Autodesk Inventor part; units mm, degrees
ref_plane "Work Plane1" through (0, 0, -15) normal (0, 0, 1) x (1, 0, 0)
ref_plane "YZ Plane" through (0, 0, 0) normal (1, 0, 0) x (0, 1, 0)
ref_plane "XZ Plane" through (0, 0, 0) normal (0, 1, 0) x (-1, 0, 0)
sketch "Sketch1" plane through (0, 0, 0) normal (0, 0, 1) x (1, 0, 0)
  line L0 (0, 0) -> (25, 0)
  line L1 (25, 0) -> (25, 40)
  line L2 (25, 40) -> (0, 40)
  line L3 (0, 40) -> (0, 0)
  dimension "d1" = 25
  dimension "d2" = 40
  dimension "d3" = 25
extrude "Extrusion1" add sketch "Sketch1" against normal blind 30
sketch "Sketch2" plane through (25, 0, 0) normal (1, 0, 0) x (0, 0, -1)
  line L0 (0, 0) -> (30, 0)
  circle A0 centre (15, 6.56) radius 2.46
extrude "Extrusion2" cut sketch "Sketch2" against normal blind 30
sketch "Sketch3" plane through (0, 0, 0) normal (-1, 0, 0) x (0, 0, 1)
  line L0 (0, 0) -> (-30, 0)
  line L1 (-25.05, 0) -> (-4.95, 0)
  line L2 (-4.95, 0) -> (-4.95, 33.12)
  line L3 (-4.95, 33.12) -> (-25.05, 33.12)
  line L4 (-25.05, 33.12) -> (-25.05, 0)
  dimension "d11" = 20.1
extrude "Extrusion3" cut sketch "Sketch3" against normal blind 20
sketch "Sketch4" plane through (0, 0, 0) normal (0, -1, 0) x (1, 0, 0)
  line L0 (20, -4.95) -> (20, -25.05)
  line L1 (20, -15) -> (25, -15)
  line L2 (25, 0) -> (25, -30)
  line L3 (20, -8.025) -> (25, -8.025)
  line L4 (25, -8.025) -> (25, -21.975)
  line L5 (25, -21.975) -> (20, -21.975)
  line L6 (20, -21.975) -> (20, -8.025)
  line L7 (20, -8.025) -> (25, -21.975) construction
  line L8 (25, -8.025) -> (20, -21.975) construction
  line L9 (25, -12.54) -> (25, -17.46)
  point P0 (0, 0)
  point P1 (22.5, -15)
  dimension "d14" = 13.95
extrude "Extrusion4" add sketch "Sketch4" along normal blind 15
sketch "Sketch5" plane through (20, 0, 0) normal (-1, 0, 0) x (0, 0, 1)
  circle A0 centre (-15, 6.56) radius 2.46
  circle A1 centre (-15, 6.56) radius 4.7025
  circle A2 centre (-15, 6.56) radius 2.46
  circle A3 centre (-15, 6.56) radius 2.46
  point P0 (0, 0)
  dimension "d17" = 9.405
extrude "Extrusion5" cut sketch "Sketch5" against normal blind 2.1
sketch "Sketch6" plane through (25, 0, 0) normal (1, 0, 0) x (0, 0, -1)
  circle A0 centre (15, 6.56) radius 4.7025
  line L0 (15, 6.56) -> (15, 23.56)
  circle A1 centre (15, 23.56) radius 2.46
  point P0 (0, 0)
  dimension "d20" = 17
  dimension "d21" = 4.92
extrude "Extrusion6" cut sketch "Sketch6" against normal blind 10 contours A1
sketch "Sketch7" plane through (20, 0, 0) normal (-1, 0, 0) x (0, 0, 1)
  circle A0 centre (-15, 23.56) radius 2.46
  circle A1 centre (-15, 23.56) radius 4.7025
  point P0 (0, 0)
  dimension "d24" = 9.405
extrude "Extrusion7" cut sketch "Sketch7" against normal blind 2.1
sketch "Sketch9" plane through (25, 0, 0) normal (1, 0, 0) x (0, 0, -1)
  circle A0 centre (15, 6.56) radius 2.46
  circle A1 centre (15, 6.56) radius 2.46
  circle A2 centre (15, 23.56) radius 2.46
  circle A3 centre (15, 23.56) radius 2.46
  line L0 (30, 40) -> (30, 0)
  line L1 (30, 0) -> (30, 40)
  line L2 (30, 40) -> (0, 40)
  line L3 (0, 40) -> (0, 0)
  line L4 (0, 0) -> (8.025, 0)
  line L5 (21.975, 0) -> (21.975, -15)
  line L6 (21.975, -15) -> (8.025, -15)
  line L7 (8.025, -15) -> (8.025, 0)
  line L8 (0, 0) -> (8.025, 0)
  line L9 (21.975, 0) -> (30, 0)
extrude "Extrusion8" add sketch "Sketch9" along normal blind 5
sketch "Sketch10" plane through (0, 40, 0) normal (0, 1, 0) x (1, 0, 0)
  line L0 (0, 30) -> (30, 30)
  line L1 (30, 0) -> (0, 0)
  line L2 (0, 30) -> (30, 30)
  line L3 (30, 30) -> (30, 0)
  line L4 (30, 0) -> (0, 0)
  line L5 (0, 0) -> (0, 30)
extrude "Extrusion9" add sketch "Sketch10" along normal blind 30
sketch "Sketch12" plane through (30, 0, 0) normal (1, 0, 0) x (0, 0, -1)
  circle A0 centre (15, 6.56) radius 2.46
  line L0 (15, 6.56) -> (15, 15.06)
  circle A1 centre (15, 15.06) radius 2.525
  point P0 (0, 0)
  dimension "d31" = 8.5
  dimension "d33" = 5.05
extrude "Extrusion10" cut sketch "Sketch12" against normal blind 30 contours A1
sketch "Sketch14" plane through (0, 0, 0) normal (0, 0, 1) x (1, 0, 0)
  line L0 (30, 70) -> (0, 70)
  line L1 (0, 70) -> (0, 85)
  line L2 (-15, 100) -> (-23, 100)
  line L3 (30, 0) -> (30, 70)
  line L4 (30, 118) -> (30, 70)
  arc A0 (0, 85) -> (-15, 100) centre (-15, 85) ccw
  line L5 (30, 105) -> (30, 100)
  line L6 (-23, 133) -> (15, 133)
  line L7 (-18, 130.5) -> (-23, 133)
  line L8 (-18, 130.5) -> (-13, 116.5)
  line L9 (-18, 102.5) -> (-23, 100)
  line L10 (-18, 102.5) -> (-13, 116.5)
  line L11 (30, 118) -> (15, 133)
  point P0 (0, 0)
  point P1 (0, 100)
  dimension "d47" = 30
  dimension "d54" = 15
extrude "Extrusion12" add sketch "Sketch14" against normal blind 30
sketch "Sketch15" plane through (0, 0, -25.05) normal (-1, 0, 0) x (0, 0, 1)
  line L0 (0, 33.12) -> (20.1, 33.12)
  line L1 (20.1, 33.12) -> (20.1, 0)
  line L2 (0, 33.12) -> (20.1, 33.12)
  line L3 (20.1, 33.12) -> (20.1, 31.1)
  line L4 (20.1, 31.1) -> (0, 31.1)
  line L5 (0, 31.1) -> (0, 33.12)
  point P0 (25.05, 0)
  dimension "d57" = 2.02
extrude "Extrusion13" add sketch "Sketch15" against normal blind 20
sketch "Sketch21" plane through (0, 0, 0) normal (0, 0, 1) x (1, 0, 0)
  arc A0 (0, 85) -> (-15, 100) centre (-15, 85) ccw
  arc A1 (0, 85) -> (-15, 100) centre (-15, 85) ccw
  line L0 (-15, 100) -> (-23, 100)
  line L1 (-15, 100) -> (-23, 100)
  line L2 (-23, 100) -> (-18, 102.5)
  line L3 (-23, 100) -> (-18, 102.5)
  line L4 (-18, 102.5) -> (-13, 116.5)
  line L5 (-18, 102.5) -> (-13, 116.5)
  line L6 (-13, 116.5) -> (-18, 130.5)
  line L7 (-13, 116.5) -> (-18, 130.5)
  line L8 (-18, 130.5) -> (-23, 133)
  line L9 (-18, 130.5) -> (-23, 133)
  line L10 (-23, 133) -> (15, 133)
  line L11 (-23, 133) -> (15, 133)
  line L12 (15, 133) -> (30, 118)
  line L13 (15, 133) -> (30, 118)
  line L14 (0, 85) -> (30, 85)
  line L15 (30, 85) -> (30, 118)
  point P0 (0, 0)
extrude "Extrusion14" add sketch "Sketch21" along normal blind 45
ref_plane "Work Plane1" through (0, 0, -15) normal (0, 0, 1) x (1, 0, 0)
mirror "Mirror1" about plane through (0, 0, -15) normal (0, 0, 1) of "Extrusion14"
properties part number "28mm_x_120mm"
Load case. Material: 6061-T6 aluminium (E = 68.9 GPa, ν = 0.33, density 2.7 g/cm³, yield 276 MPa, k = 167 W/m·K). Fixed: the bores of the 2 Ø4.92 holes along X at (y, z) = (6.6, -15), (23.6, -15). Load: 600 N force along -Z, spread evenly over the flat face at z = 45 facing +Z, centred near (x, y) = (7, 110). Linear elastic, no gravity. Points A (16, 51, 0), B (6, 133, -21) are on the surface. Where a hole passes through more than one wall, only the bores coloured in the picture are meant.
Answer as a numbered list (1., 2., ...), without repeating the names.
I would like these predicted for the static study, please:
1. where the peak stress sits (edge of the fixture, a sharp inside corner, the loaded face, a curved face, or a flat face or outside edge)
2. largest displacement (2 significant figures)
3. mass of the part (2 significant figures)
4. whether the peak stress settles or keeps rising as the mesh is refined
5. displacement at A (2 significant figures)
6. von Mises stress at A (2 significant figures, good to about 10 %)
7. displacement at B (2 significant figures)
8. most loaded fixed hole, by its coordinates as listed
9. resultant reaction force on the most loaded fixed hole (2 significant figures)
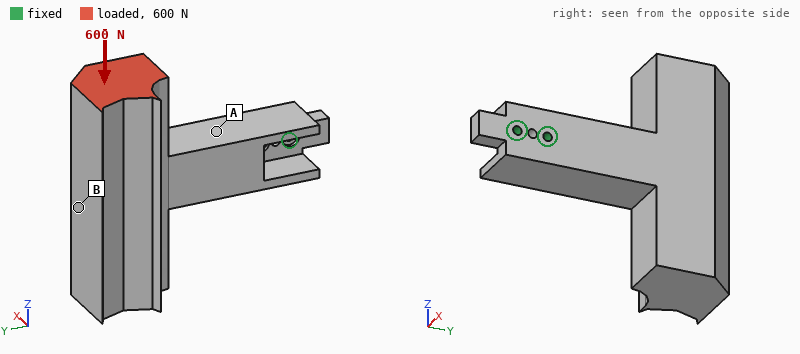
1. edge of the fixture
2. 0.15 mm
3. 800 g
4. keeps rising
5. 0.029 mm
6. 8.5 MPa
7. 0.12 mm
8. (23.6, -15)
9. 2.8 kN
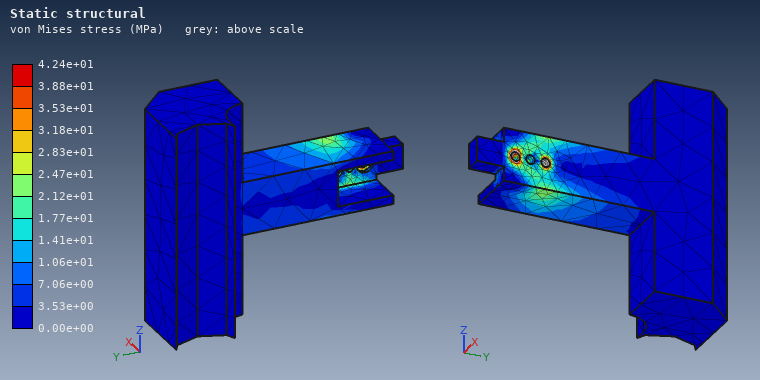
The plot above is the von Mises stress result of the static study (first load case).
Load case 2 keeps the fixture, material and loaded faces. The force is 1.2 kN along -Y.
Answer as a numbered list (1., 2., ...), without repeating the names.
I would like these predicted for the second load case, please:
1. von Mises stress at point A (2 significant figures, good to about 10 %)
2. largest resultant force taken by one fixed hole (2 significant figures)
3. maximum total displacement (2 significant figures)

1. 18 MPa
2. 3.3 kN
3. 0.25 mm
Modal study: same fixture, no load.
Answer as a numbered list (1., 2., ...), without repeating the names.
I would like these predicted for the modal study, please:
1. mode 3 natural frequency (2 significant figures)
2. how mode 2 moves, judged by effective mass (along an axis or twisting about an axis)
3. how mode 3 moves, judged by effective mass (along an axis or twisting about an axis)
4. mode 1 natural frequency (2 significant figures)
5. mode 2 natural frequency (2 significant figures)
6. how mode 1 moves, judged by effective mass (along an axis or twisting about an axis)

1. 670 Hz
2. along Z
3. twisting about Y
4. 420 Hz
5. 450 Hz
6. along X
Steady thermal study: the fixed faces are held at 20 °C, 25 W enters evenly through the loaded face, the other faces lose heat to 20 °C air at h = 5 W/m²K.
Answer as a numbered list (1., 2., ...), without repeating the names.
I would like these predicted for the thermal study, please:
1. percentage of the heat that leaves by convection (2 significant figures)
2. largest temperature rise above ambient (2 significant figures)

1. 9.3 %
2. 19 K
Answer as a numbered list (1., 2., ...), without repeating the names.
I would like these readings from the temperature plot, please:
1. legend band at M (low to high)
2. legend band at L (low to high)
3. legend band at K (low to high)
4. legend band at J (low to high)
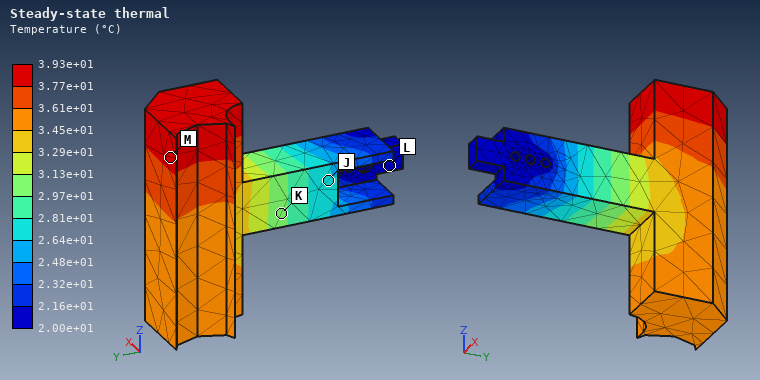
1. 3.77e+01 to 3.93e+01 °C
2. 2.00e+01 to 2.16e+01 °C
3. 2.97e+01 to 3.13e+01 °C
4. 2.64e+01 to 2.81e+01 °C
